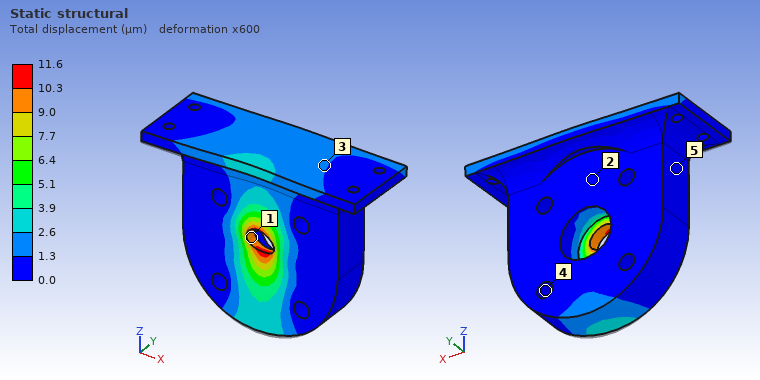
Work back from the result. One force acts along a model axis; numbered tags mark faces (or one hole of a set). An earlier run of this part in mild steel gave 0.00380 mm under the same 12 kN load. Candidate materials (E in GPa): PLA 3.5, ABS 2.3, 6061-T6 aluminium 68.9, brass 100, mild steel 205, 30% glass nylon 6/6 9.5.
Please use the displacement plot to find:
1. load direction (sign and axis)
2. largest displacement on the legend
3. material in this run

+Z
11.6 µm
6061-T6 aluminium
